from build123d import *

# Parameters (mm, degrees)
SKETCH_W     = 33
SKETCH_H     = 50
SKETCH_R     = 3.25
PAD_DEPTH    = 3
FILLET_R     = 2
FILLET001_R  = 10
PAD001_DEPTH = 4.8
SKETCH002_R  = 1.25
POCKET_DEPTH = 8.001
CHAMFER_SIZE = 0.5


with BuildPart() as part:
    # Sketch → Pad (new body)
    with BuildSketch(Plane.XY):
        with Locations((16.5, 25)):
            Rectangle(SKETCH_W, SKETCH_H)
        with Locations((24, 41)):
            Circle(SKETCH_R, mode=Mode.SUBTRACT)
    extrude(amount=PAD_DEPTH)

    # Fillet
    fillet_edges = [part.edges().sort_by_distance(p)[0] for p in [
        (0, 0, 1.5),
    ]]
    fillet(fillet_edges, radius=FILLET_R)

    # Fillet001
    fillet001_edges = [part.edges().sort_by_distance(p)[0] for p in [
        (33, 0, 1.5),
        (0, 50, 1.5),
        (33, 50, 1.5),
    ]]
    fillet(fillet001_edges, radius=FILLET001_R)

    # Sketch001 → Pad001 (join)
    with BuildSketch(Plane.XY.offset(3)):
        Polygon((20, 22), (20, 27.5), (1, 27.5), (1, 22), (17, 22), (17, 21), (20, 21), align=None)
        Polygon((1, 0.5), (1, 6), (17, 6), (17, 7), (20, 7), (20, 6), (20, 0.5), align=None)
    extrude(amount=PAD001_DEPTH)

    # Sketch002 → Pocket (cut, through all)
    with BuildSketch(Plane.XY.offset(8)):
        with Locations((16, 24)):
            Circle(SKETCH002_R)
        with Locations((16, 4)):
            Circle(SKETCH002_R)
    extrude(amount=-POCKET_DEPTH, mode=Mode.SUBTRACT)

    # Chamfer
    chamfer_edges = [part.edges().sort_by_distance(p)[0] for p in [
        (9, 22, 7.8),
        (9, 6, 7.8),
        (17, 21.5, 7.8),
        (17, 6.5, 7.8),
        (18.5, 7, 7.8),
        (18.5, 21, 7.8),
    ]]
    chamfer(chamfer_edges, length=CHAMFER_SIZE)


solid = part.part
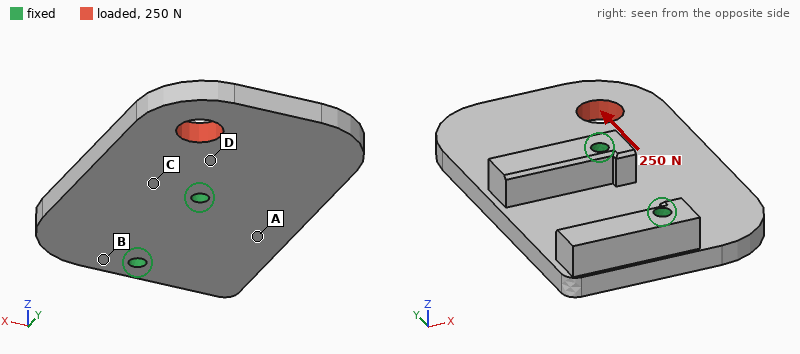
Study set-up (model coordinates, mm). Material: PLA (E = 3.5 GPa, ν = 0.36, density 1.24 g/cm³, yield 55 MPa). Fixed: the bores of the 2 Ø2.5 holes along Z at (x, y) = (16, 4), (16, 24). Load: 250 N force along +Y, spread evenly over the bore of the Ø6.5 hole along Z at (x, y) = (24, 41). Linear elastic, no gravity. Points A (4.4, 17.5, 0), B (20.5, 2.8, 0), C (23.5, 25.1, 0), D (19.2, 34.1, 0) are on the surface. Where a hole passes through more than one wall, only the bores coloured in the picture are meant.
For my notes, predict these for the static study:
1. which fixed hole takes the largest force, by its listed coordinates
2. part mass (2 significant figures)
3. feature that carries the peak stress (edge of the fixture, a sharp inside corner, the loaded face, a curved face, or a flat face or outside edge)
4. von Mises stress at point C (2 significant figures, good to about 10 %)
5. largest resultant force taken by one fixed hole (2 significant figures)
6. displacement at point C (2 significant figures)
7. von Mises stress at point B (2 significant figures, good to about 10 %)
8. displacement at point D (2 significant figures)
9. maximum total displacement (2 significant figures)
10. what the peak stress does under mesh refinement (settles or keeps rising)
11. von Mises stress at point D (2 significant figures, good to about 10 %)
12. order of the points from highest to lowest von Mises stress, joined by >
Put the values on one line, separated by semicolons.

(16, 24); 7.0 g; edge of the fixture; 4.1 MPa; 210 N; 22 µm; 2.2 MPa; 30 µm; 77 µm; keeps rising; 5.1 MPa; D > C > B > A
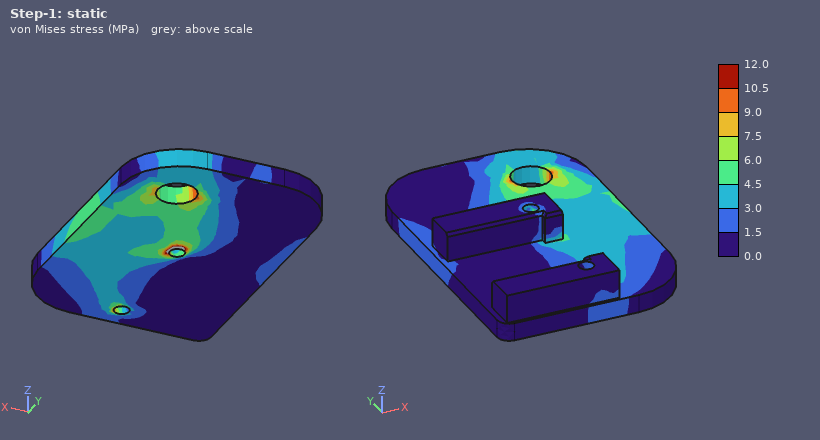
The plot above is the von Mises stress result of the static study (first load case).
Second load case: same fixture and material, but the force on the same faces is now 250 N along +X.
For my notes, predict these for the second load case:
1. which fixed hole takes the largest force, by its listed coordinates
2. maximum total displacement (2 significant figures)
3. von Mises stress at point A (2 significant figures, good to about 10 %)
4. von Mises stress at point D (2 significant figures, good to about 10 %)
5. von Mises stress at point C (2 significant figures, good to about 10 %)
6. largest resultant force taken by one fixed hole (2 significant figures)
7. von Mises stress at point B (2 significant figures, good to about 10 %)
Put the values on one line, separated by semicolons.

(16, 24); 0.17 mm; 4.1 MPa; 6.3 MPa; 5.4 MPa; 430 N; 3.0 MPa
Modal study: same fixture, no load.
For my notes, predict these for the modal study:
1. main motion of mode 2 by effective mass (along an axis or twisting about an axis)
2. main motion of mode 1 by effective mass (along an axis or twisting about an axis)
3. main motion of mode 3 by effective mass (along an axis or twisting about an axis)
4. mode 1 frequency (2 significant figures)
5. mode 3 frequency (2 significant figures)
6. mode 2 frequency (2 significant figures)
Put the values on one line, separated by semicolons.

twisting about Y; along Z; along Z; 1400 Hz; 3800 Hz; 2300 Hz
